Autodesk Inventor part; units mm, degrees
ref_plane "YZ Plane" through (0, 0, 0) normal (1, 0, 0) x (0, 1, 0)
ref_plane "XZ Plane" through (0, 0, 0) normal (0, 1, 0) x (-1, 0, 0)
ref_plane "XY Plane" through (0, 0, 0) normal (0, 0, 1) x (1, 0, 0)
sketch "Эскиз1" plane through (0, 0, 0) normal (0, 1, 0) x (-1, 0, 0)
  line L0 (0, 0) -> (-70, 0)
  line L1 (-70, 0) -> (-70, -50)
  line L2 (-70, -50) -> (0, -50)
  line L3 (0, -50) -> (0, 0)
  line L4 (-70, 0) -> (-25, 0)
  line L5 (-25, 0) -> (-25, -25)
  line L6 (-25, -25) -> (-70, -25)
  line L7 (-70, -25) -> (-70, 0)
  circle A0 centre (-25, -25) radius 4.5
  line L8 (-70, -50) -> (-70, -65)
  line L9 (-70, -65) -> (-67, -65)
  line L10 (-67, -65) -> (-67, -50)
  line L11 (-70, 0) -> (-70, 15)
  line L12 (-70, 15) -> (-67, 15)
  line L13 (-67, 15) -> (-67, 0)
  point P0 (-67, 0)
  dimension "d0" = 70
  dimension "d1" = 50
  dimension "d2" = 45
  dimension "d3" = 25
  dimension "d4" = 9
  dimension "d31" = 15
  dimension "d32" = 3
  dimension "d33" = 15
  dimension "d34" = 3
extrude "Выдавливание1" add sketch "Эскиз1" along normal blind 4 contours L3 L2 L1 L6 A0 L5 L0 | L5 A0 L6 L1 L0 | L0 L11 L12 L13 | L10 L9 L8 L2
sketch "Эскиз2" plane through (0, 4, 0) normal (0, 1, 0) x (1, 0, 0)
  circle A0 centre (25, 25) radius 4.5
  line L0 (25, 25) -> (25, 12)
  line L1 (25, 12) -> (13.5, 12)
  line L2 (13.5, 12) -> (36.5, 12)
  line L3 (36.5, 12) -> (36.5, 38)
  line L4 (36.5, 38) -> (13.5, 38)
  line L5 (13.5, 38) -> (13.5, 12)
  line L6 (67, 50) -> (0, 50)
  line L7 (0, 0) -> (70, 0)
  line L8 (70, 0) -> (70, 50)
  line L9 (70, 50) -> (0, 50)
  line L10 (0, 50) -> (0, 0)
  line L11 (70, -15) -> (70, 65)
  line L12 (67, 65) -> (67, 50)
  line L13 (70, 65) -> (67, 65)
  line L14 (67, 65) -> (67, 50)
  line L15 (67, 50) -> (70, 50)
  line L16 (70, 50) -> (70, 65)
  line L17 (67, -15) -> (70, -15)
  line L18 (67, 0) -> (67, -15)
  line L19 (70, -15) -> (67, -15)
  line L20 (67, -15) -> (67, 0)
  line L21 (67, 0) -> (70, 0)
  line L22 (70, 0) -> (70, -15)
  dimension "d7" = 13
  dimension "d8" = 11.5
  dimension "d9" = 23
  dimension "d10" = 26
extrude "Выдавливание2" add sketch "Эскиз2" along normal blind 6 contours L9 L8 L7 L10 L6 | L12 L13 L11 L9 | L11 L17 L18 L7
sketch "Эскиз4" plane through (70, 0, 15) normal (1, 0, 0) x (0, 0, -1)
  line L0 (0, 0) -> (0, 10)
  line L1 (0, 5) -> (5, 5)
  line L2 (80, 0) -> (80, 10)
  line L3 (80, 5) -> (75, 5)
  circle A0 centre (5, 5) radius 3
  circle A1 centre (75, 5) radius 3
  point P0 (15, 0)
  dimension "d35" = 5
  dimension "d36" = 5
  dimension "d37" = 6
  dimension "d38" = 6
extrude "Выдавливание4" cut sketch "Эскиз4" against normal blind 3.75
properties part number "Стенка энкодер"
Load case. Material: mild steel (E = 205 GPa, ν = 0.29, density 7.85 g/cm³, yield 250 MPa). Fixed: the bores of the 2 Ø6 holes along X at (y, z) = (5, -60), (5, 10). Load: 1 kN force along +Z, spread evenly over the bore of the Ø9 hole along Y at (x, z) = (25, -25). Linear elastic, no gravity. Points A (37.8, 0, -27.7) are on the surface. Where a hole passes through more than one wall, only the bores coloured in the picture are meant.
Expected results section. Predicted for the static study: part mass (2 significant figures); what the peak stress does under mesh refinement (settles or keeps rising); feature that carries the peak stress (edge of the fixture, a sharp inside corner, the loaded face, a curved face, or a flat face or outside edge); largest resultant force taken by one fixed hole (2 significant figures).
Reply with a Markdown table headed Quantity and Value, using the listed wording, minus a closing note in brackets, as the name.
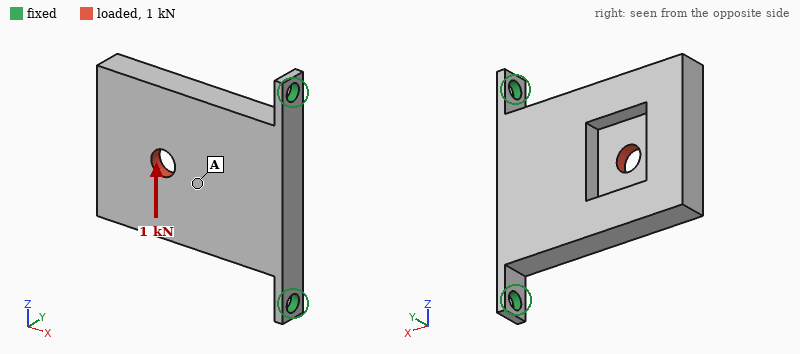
| Quantity | Value |
|---|---|
| part mass | 250 g |
| what the peak stress does under mesh refinement | keeps rising |
| feature that carries the peak stress | edge of the fixture |
| largest resultant force taken by one fixed hole | 920 N |
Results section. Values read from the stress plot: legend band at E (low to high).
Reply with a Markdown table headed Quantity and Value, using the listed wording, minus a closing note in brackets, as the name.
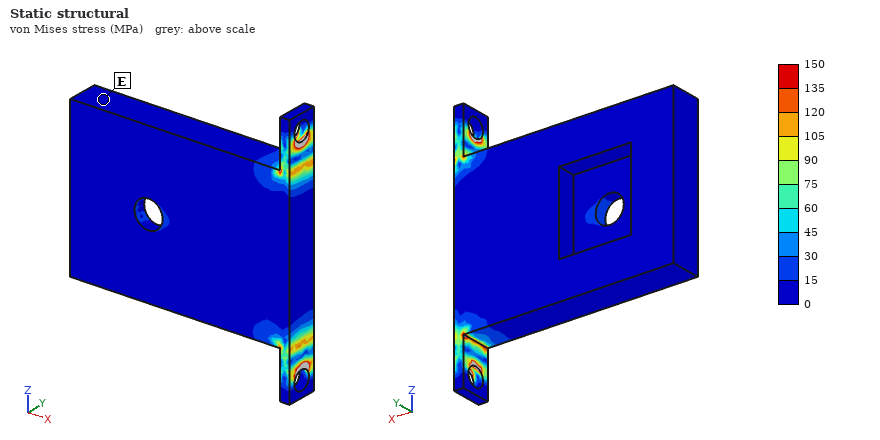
| Quantity | Value |
|---|---|
| legend band at E | 0 to 15 MPa |
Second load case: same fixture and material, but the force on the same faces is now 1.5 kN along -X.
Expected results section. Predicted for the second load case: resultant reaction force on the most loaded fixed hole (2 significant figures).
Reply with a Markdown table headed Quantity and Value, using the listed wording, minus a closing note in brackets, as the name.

| Quantity | Value |
|---|---|
| resultant reaction force on the most loaded fixed hole | 880 N |
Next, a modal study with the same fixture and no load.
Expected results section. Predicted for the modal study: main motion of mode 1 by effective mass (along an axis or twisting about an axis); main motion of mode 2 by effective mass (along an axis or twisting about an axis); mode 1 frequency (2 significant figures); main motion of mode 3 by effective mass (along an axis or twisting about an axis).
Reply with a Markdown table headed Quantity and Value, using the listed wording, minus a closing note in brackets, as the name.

| Quantity | Value |
|---|---|
| main motion of mode 1 by effective mass | along Y |
| main motion of mode 2 by effective mass | along Z |
| mode 1 frequency | 340 Hz |
| main motion of mode 3 by effective mass | along X |
